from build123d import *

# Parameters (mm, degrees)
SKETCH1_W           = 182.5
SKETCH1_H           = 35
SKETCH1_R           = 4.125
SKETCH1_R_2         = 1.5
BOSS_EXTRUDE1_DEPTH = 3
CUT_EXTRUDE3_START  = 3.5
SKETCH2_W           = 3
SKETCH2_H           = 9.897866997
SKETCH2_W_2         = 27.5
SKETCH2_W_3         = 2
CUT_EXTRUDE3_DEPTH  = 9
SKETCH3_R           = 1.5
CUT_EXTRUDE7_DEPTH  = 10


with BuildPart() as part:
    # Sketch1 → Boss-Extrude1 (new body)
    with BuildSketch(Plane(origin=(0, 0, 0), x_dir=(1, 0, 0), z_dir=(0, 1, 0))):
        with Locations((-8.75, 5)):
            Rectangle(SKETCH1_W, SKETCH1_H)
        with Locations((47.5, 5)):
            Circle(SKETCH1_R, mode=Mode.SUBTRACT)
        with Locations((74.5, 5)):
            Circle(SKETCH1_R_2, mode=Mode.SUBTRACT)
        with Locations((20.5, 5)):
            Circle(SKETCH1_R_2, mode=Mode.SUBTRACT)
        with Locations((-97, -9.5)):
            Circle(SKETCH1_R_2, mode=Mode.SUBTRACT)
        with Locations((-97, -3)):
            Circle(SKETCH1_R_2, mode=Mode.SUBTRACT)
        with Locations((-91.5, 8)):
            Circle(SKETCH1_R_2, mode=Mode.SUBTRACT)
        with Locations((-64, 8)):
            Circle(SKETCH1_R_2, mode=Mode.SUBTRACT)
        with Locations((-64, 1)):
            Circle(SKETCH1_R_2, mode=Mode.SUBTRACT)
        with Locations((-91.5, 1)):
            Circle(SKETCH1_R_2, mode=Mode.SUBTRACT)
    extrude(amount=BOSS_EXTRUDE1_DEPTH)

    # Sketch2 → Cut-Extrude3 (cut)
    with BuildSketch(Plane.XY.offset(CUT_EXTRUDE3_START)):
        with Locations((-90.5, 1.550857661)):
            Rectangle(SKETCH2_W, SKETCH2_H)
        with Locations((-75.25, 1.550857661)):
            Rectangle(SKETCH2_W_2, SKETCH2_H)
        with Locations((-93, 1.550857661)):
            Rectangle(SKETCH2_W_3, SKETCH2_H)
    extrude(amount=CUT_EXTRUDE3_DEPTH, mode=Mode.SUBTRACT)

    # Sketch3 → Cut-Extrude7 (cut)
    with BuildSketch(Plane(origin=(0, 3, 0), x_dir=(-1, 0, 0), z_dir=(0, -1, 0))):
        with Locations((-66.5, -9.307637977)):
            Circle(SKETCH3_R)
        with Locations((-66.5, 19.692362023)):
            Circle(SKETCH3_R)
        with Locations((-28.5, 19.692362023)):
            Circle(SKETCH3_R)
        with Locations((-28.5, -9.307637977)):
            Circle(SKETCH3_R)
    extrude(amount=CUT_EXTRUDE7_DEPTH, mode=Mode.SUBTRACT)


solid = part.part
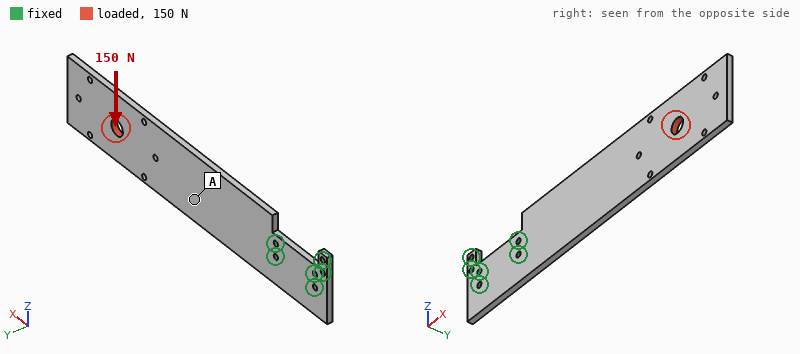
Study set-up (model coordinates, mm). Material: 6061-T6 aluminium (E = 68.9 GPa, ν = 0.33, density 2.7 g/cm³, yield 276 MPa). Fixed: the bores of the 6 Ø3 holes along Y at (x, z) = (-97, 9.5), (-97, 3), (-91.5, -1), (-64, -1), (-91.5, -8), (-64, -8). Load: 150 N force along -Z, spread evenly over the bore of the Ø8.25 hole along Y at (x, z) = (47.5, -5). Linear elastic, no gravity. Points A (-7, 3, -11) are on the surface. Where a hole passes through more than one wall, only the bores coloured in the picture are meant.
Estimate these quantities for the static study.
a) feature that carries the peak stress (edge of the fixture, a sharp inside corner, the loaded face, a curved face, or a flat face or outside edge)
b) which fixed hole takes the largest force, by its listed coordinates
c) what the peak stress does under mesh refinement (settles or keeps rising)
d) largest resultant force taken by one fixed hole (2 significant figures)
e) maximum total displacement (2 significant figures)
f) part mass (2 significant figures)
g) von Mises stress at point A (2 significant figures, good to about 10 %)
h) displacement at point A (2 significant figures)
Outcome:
edge of the fixture
(-64, -1)
keeps rising
980 N
0.26 mm
48 g
5.5 MPa
0.076 mm
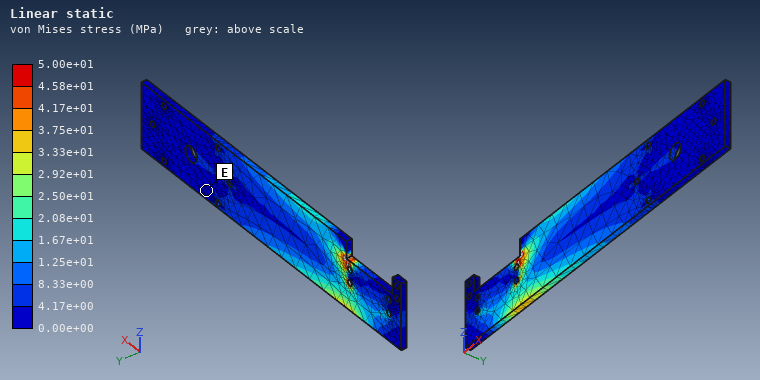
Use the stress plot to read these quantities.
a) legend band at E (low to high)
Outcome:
0.00e+00 to 4.17e+00 MPa
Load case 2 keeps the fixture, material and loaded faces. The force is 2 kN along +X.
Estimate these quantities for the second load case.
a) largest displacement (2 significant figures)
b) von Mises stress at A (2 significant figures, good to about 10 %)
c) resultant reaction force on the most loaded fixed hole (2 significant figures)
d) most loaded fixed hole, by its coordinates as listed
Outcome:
51 µm
19 MPa
1.0 kN
(-64, -1)
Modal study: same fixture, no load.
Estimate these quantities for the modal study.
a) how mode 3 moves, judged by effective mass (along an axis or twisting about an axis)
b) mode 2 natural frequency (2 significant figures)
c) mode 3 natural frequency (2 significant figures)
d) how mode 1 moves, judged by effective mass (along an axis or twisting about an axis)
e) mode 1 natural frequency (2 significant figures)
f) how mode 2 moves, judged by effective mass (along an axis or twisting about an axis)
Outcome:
twisting about X
700 Hz
890 Hz
along Y
110 Hz
along Y
